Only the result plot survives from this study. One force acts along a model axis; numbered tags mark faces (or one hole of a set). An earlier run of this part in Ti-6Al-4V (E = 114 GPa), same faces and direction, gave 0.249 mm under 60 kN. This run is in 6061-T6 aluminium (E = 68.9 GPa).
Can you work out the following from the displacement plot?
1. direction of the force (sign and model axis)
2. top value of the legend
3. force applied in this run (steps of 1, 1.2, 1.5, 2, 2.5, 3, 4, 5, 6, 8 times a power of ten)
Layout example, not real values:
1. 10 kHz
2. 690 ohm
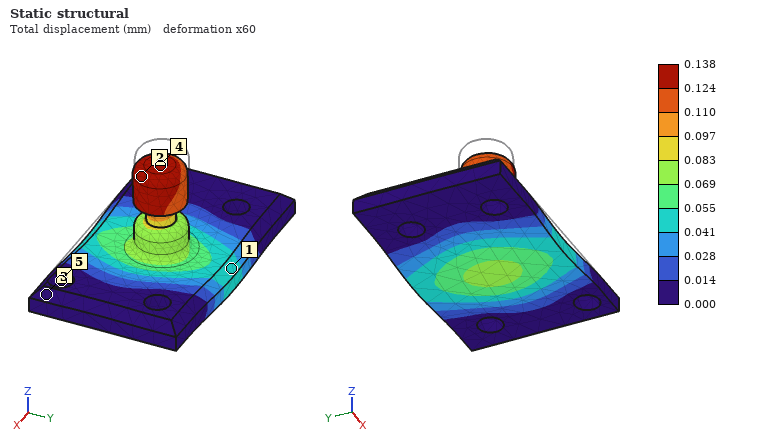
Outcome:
1. -Z
2. 0.138 mm
3. 20 kN
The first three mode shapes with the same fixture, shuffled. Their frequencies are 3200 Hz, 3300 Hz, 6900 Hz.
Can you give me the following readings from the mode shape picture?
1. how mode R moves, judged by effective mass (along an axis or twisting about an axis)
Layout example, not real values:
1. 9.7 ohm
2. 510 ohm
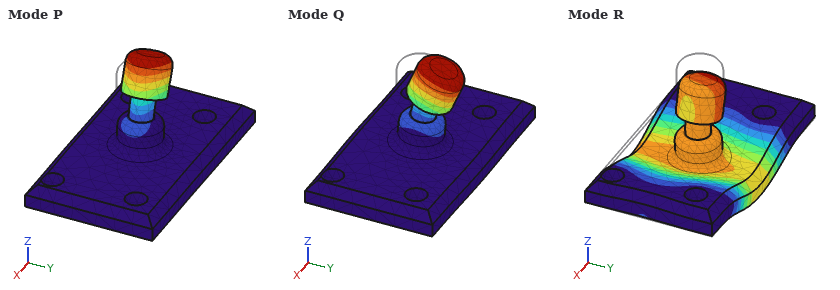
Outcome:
1. along Z
